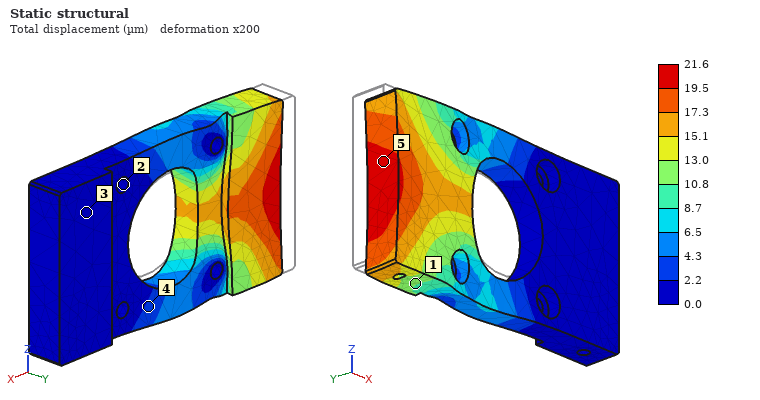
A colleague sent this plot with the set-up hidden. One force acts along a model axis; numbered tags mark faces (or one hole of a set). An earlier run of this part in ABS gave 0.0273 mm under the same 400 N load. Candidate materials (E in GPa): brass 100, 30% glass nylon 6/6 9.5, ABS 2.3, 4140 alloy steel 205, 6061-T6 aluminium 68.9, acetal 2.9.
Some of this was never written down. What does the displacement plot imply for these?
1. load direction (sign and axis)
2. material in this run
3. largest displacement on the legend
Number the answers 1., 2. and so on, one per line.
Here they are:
1. +X
2. acetal
3. 21.6 µm
